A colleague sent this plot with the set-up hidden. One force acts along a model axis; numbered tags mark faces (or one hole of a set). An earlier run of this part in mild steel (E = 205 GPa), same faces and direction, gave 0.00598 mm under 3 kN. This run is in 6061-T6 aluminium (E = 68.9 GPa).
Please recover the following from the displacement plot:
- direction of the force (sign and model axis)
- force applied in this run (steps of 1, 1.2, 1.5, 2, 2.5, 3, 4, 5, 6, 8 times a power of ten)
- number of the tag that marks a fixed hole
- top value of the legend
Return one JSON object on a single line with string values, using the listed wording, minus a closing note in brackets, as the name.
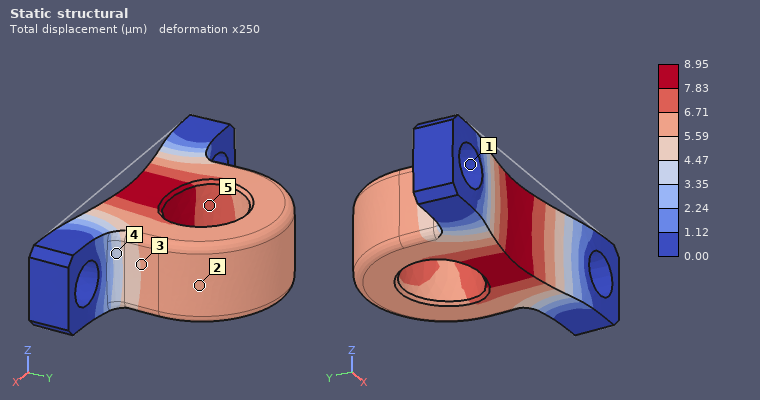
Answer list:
{"direction of the force": "+Y", "force applied in this run": "1.5 kN", "number of the tag that marks a fixed hole": "1", "top value of the legend": "8.95 µm"}
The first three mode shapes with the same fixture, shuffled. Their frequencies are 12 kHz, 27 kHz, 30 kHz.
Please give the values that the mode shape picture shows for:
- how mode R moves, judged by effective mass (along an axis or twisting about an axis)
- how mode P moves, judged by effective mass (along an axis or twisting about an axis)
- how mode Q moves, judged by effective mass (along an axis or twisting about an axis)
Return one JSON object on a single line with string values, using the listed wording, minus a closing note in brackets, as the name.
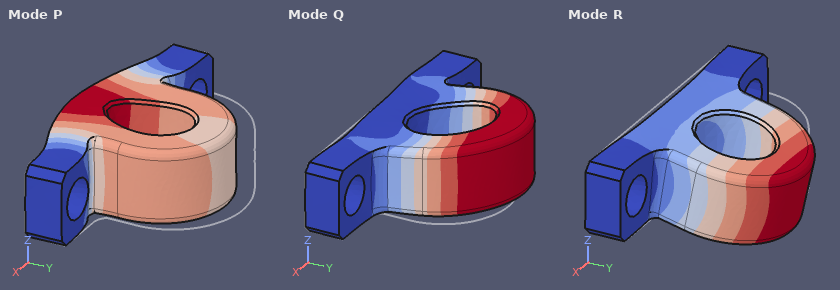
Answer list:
{"how mode R moves, judged by effective mass": "along Z", "how mode P moves, judged by effective mass": "along Y", "how mode Q moves, judged by effective mass": "along X"}
